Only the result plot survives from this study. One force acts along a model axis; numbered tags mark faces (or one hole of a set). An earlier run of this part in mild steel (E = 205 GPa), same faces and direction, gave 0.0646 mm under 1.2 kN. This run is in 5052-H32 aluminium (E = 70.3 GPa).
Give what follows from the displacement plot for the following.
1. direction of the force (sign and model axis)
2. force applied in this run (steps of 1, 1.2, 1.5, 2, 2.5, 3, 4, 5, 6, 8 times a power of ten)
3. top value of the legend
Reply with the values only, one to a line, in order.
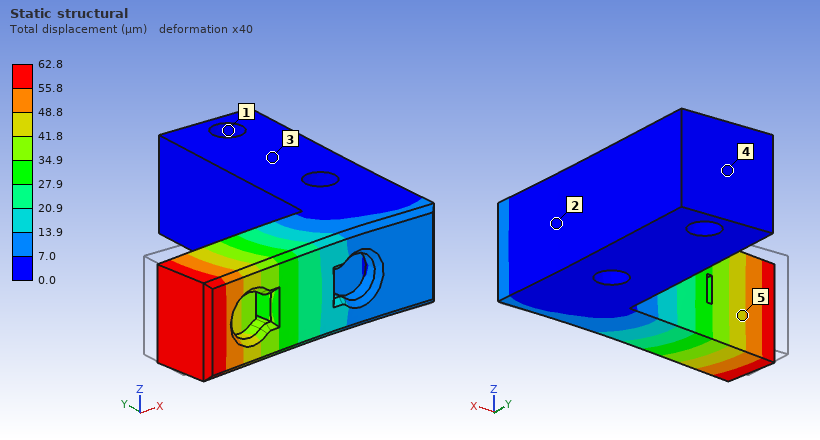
-Y
400 N
62.8 µm
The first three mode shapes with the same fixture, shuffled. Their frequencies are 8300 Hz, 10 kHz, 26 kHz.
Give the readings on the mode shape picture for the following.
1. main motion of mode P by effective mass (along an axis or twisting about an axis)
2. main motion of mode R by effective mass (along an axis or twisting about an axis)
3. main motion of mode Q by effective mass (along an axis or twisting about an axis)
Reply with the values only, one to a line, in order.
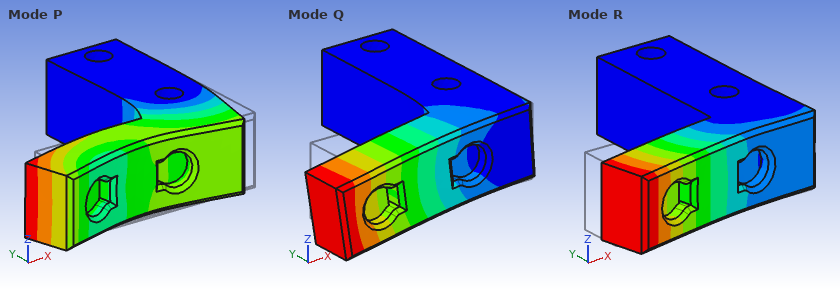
along X
along Y
along Z
